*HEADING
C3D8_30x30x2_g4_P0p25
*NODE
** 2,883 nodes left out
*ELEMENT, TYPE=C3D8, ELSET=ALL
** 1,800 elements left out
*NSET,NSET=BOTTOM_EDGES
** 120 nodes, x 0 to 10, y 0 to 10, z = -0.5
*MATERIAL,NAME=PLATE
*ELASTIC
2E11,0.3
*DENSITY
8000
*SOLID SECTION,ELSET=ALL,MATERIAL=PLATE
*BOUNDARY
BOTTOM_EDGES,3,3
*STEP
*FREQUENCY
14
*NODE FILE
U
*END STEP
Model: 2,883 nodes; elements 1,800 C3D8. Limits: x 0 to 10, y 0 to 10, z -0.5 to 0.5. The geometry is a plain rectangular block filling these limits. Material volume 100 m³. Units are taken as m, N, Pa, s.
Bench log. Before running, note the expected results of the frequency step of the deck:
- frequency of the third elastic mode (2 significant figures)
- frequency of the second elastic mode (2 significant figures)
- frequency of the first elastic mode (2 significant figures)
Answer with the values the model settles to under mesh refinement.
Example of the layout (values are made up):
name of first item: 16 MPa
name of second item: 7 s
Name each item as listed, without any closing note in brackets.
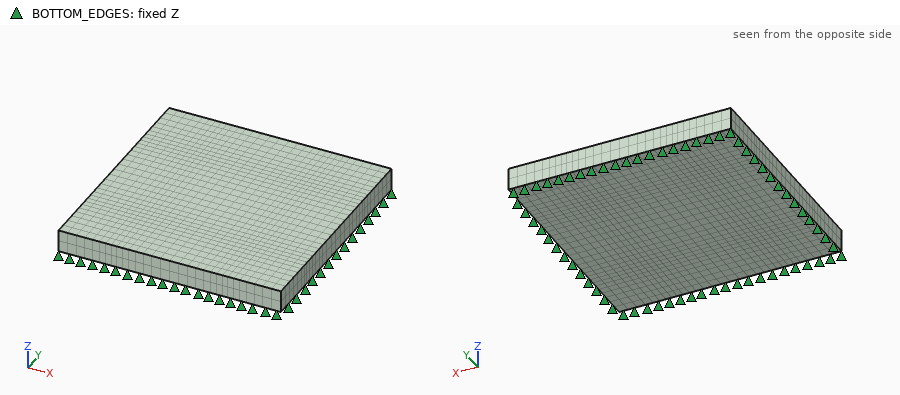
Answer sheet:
frequency of the third elastic mode: 100 Hz
frequency of the second elastic mode: 100 Hz
frequency of the first elastic mode: 43 Hz
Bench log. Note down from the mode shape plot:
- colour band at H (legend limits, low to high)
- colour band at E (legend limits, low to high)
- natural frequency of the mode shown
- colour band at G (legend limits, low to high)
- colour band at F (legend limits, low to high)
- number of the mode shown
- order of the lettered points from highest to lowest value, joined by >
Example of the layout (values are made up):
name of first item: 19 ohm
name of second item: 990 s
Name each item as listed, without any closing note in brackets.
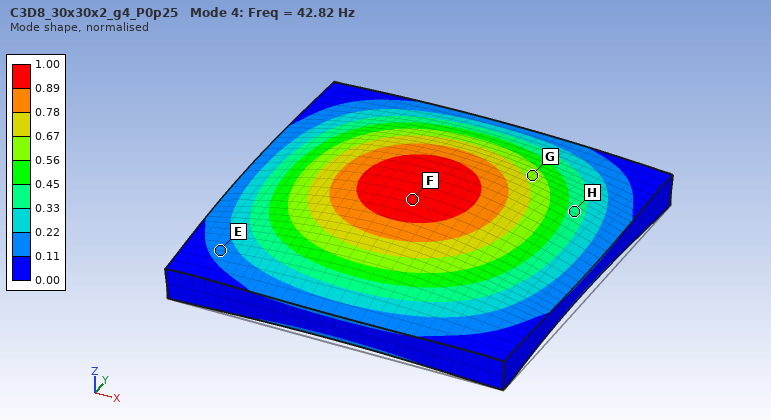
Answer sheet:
colour band at H: 0.33 to 0.45
colour band at E: 0.11 to 0.22
natural frequency of the mode shown: 42.82 Hz
colour band at G: 0.56 to 0.67
colour band at F: 0.89 to 1.00
number of the mode shown: 4
order of the lettered points from highest to lowest value, joined by >: F > G > H > E
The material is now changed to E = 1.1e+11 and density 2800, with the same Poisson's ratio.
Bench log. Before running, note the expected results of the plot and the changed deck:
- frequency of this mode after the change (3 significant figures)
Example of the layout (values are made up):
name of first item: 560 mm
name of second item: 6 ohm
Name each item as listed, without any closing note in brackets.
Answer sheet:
frequency of this mode after the change: 53.7 Hz
